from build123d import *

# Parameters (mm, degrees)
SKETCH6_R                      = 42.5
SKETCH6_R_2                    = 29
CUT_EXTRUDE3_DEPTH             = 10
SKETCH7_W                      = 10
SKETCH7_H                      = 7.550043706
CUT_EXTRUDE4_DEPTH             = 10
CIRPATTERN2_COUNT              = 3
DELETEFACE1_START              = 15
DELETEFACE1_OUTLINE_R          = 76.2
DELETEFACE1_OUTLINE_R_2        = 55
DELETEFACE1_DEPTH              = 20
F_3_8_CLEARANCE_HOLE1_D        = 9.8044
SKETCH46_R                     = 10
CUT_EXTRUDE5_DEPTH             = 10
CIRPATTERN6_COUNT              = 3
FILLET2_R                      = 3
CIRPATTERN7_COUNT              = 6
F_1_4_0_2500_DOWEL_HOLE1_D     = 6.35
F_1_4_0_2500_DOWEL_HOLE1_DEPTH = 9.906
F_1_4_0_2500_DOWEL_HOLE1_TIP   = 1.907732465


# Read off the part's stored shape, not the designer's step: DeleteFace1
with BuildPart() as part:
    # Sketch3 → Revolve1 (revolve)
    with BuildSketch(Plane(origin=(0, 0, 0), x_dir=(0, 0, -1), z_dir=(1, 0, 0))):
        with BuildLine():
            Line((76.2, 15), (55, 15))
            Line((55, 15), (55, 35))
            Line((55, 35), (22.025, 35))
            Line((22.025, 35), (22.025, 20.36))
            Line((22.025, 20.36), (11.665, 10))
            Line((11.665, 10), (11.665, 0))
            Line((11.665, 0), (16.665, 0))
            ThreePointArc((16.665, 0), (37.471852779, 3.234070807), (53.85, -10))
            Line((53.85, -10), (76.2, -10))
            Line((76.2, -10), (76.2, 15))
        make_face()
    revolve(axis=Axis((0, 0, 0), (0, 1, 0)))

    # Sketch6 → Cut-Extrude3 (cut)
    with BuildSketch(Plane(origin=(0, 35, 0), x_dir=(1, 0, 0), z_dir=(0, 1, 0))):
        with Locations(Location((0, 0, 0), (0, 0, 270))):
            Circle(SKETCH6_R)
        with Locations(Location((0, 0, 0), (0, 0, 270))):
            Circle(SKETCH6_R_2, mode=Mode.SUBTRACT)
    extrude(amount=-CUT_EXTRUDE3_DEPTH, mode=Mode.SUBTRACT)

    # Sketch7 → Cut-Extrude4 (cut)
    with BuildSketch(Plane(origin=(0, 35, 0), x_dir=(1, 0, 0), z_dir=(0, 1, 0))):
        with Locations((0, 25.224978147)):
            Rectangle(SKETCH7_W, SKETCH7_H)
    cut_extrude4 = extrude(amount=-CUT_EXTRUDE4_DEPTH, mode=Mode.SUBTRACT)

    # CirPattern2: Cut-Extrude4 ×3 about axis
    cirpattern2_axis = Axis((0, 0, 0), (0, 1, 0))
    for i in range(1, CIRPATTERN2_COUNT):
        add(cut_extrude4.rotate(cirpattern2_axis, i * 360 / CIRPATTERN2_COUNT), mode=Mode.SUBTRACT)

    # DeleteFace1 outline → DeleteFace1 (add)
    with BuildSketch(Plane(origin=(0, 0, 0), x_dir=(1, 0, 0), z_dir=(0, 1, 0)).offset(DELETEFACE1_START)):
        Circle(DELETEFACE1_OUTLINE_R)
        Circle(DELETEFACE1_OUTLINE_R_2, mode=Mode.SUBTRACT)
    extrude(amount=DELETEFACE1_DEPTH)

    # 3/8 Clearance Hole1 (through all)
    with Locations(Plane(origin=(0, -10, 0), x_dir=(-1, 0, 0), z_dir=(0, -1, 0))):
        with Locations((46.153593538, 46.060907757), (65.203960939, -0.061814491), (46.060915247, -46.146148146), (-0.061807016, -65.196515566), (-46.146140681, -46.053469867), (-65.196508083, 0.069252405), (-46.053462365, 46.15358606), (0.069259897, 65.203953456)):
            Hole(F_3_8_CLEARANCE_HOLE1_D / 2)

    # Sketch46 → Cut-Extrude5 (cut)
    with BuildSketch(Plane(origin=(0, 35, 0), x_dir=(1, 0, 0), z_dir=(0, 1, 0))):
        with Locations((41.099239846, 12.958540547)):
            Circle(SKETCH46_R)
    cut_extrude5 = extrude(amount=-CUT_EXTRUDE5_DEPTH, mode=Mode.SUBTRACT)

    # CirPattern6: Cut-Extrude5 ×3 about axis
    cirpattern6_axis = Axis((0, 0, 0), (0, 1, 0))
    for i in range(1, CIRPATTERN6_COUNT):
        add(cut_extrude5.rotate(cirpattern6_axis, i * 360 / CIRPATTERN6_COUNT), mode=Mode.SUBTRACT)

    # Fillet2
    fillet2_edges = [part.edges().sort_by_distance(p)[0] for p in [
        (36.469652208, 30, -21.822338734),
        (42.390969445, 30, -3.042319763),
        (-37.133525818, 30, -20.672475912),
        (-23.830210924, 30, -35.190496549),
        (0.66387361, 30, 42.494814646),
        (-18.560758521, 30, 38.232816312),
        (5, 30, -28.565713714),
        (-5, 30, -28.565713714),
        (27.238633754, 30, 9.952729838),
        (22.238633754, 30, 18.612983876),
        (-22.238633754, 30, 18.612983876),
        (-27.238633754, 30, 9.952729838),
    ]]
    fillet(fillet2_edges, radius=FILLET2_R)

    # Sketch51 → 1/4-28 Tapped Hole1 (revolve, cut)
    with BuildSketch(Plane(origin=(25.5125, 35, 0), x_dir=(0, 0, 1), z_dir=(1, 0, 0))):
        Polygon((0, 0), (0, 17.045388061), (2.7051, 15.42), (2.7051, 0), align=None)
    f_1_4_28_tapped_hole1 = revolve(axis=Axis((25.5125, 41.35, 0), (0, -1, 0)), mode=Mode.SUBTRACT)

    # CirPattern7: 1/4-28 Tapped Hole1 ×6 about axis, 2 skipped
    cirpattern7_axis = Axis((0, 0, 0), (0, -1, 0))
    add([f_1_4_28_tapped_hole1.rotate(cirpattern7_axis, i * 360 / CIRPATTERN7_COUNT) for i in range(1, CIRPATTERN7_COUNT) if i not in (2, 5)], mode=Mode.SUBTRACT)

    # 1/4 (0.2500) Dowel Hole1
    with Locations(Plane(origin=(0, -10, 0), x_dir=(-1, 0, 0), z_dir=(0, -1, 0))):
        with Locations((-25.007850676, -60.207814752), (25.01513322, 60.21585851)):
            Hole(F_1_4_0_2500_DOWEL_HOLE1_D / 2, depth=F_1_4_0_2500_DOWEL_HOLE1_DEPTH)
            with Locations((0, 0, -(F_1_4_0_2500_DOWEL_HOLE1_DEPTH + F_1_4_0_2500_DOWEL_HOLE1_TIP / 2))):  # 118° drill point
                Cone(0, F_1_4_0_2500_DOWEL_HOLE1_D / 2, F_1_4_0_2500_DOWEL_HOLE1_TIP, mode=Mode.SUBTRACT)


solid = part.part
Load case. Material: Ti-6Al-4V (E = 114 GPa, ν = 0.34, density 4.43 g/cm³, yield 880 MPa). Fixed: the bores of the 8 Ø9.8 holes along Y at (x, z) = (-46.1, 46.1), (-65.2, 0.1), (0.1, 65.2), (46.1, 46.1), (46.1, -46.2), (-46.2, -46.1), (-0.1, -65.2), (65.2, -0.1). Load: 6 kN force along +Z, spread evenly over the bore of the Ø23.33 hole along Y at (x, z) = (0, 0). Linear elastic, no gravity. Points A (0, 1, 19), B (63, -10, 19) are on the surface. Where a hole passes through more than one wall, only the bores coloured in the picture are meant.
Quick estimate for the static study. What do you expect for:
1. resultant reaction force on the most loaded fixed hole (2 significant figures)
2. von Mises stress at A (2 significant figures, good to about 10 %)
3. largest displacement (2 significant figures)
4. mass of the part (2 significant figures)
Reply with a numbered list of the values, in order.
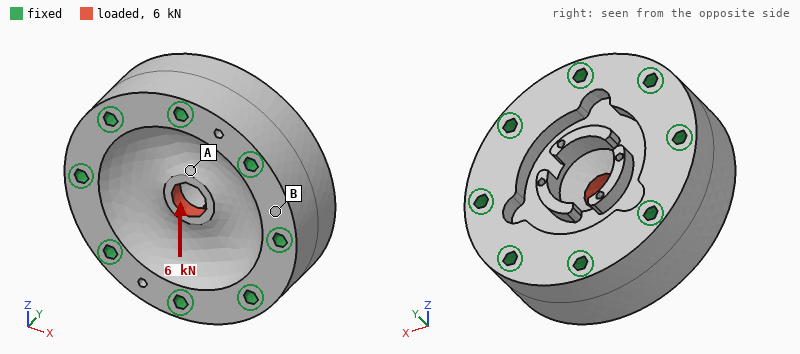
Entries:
1. 1.3 kN
2. 8.9 MPa
3. 2.6 µm
4. 2.8 kg
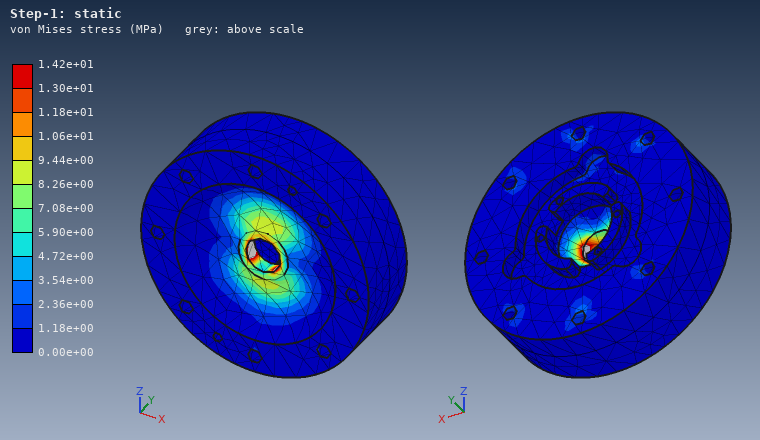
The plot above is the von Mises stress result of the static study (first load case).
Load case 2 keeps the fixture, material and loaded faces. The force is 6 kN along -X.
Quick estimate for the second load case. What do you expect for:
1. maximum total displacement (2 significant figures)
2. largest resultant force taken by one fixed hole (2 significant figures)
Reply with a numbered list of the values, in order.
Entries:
1. 2.6 µm
2. 1.3 kN
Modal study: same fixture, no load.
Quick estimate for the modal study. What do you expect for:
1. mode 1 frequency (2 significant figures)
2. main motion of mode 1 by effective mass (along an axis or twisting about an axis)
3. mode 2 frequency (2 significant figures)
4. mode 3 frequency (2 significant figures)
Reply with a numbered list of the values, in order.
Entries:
1. 14 kHz
2. along Y
3. 19 kHz
4. 19 kHz
